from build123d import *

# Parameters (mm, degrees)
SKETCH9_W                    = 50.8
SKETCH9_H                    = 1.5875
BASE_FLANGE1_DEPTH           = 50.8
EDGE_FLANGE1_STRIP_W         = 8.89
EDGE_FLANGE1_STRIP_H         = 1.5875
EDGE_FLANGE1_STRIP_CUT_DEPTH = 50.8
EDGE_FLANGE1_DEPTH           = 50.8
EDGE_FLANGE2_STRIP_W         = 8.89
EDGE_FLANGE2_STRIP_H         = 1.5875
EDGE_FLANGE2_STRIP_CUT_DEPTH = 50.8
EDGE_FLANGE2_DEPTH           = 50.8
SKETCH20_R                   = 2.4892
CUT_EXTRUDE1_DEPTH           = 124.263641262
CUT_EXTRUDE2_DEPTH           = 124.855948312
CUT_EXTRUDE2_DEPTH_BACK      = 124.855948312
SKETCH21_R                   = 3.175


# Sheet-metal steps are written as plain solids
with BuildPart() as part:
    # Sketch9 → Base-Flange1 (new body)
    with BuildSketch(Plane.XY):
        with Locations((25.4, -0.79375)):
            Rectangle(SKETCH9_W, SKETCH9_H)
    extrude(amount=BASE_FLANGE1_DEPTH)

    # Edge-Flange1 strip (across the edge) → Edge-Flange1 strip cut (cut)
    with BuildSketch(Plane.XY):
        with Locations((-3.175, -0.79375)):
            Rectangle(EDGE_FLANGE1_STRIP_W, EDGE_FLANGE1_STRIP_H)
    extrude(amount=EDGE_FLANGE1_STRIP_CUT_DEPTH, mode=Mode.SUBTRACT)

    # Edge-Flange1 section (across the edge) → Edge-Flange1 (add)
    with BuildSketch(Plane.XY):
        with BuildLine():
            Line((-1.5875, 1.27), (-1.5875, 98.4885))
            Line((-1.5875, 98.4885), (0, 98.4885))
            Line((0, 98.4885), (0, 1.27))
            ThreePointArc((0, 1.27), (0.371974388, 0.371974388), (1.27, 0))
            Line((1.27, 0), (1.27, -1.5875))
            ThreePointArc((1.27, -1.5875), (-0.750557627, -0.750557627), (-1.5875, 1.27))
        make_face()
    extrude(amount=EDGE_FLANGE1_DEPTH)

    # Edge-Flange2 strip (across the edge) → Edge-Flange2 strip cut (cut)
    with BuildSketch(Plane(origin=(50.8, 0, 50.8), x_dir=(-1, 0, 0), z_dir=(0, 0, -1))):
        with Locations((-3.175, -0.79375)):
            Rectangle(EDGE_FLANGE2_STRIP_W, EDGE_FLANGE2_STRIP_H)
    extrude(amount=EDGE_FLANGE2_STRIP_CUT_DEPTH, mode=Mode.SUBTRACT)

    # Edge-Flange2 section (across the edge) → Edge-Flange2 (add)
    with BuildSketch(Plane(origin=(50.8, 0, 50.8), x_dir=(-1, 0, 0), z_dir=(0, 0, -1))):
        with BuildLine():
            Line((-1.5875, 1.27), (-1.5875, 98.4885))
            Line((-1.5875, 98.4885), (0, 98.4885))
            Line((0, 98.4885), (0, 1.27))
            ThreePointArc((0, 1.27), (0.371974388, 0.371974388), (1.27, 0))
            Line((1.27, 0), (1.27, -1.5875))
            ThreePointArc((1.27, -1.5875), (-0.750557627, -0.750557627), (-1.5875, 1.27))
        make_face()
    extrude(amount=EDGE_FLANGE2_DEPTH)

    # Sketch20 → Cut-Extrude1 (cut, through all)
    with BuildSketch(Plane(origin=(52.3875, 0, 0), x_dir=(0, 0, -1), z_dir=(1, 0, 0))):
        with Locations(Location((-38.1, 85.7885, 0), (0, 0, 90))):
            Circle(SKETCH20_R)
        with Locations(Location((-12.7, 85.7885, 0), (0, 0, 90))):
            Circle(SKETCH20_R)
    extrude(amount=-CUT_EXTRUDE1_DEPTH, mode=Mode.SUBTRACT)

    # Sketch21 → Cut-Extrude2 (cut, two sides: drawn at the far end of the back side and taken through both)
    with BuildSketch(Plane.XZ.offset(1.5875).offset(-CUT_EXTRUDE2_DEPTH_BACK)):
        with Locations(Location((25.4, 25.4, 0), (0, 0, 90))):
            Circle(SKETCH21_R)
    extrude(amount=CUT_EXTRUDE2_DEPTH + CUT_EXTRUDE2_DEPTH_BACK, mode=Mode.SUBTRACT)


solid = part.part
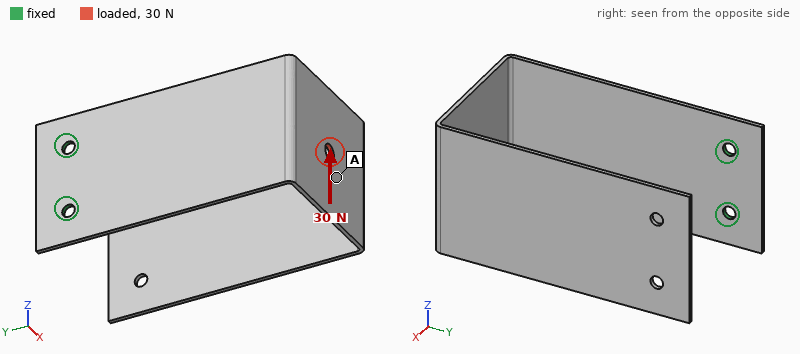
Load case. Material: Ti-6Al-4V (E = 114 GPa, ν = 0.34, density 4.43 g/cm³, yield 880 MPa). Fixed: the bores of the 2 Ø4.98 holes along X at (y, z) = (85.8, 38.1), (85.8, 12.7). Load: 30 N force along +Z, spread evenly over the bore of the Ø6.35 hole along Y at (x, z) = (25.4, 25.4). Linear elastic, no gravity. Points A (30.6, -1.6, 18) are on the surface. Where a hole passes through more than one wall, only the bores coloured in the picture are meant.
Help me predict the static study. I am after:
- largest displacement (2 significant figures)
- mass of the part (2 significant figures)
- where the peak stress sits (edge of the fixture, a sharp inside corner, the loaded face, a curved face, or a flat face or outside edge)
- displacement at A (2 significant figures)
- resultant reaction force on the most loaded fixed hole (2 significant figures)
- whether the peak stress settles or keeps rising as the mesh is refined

1.3 mm
88 g
edge of the fixture
0.61 mm
96 N
keeps rising
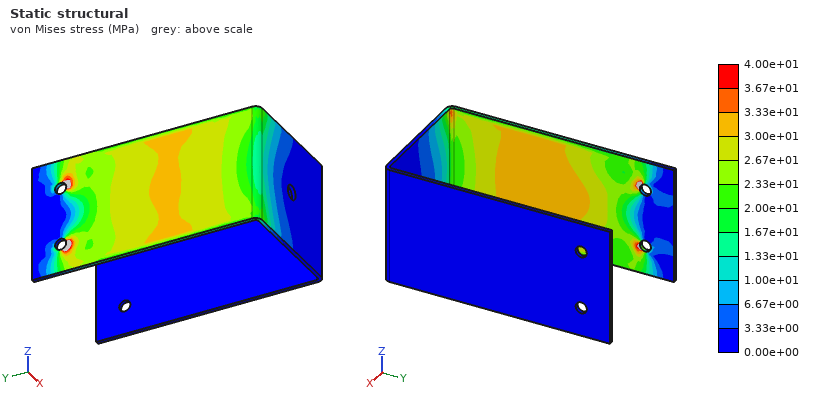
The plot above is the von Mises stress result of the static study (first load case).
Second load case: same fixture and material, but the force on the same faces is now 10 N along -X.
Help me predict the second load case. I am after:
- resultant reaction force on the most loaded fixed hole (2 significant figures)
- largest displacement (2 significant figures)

5.0 N
1.4 mm
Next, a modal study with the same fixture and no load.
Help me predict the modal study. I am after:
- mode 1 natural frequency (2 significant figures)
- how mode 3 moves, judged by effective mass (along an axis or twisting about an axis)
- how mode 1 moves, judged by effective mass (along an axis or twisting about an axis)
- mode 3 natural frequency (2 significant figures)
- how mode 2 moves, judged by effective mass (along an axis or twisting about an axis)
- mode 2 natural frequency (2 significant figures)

50 Hz
along X
along Y
78 Hz
along Z
73 Hz
